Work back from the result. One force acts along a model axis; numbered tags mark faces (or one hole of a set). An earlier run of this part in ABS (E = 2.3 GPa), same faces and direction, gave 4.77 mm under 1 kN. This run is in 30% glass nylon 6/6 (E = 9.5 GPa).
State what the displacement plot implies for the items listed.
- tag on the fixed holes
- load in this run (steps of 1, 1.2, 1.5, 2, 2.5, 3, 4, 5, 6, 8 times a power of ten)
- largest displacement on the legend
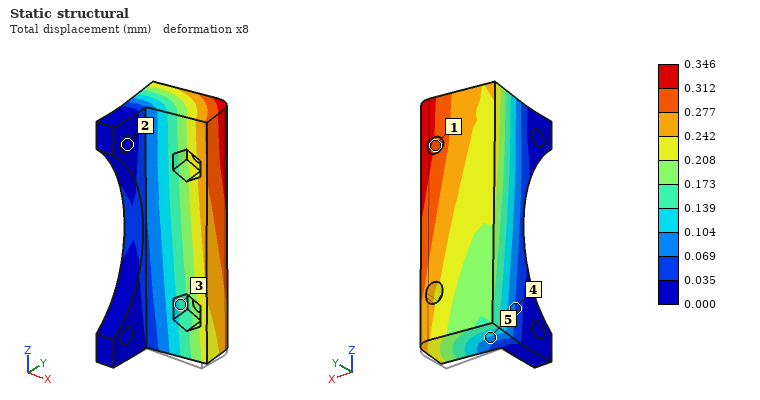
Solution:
2
300 N
0.346 mm
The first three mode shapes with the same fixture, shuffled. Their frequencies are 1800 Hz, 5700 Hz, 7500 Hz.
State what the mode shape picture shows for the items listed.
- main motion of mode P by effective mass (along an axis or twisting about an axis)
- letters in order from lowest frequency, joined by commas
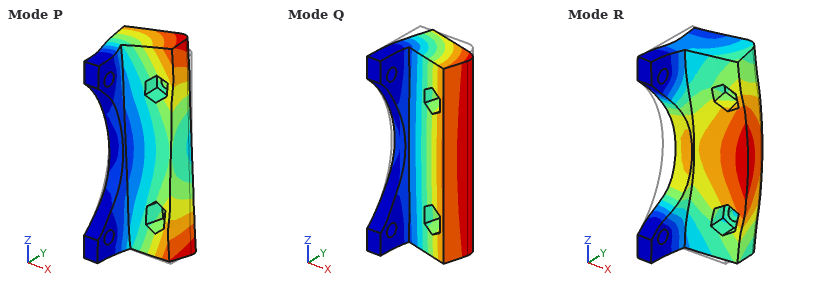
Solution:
along Z
Q, P, R
